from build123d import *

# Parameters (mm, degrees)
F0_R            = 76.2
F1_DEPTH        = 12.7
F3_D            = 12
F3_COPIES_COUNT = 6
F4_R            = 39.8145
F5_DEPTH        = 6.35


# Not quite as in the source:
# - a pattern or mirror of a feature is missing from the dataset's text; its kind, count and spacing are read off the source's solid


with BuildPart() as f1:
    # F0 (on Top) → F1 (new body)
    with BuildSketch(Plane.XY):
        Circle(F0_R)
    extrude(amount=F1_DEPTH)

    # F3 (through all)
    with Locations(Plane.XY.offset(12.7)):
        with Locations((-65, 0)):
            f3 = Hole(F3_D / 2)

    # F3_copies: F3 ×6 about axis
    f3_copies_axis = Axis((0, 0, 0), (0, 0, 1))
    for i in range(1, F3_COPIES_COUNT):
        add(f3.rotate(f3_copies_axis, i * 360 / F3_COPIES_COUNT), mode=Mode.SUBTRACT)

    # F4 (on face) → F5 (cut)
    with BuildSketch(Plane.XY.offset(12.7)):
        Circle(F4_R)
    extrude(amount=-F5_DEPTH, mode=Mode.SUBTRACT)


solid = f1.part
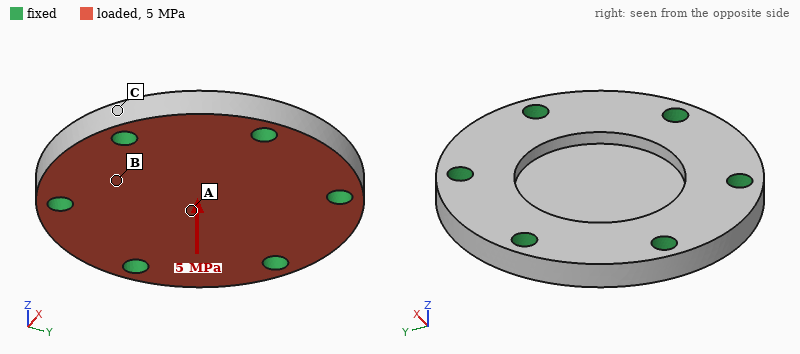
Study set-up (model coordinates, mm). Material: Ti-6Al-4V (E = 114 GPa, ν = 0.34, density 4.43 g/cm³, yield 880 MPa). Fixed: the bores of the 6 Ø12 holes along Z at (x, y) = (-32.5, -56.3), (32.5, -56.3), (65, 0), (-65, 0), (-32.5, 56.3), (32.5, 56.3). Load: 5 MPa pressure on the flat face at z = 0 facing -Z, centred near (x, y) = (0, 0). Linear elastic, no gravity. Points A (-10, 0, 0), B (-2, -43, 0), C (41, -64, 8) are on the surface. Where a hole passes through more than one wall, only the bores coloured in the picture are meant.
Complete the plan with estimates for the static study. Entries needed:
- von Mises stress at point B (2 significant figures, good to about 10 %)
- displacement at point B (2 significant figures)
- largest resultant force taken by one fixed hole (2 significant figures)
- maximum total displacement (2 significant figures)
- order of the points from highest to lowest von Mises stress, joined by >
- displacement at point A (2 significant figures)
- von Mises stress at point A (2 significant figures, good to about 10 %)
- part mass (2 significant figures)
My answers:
77 MPa
0.045 mm
15 kN
0.18 mm
A > B > C
0.17 mm
140 MPa
850 g
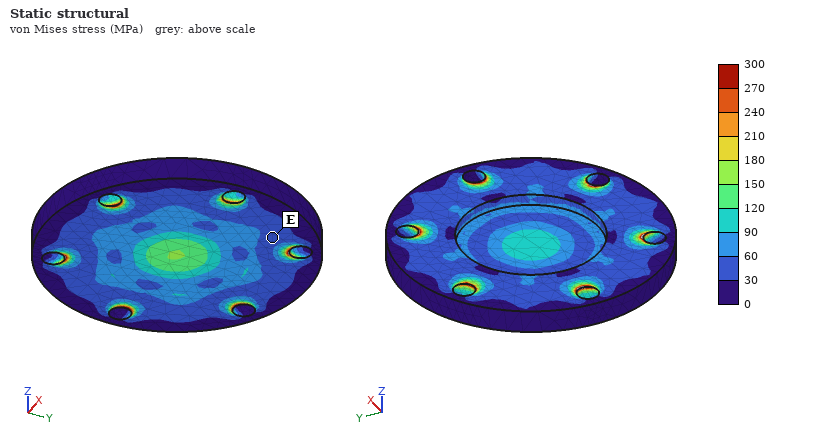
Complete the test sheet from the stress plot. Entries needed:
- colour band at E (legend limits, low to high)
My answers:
30 to 60 MPa
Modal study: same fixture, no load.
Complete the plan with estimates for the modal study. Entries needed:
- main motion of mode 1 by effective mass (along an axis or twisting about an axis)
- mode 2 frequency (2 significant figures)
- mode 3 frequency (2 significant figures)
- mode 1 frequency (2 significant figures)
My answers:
along Z
10 kHz
10 kHz
6200 Hz
